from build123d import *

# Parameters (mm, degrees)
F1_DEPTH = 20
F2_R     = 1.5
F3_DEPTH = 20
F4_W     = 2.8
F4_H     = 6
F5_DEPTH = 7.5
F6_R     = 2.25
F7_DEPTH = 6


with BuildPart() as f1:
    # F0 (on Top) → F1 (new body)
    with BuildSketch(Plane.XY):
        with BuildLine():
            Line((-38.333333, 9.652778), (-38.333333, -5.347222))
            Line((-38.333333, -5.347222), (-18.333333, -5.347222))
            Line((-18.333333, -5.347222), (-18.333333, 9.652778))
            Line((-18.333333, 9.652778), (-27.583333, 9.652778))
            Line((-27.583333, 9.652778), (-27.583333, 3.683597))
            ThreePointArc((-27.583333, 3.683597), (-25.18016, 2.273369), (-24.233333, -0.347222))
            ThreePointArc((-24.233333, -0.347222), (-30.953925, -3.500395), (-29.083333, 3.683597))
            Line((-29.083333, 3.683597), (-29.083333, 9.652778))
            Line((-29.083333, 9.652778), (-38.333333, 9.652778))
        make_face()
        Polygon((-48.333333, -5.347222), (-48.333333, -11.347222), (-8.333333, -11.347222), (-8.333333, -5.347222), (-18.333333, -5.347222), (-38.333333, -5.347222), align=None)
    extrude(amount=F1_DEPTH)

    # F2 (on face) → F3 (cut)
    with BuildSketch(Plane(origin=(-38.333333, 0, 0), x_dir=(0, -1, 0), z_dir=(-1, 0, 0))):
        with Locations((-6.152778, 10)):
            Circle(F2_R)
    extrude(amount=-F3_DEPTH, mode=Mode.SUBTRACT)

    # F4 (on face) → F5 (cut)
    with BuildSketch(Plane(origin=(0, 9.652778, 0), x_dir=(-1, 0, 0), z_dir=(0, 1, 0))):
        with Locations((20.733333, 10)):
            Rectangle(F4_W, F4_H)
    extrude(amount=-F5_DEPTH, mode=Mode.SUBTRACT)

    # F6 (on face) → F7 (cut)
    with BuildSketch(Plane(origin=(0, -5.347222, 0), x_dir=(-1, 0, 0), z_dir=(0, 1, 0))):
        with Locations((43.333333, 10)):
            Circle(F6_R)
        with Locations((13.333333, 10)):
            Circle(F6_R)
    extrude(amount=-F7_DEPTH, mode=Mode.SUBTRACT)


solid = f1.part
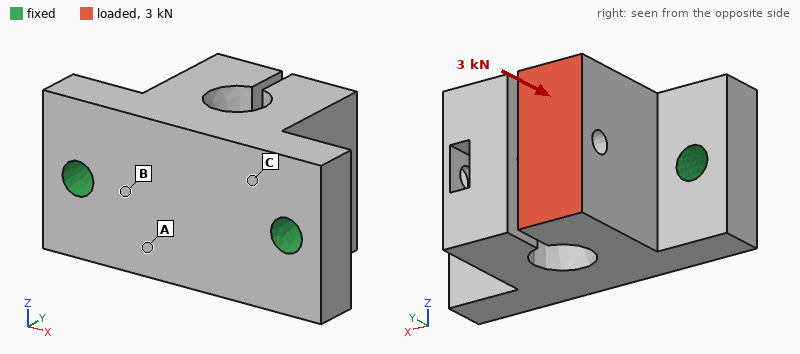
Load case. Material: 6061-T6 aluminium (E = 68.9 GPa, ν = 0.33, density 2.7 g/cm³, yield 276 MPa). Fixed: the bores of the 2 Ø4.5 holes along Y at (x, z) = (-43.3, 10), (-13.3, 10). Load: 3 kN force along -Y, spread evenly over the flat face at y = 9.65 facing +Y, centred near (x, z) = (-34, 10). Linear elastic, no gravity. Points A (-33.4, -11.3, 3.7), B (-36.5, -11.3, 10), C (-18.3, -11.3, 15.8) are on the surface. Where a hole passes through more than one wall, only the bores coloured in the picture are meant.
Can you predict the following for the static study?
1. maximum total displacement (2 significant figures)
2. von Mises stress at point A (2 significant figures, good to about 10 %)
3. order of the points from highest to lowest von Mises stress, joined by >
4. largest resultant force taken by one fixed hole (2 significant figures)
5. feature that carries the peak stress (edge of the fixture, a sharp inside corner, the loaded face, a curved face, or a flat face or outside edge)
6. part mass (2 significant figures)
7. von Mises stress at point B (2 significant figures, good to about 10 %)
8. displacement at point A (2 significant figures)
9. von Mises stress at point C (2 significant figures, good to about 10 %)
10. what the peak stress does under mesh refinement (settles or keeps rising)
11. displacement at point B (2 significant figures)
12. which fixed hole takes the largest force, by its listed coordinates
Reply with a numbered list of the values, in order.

1. 41 µm
2. 37 MPa
3. A > B > C
4. 2.2 kN
5. edge of the fixture
6. 25 g
7. 21 MPa
8. 13 µm
9. 11 MPa
10. keeps rising
11. 9.8 µm
12. (-43.3, 10)
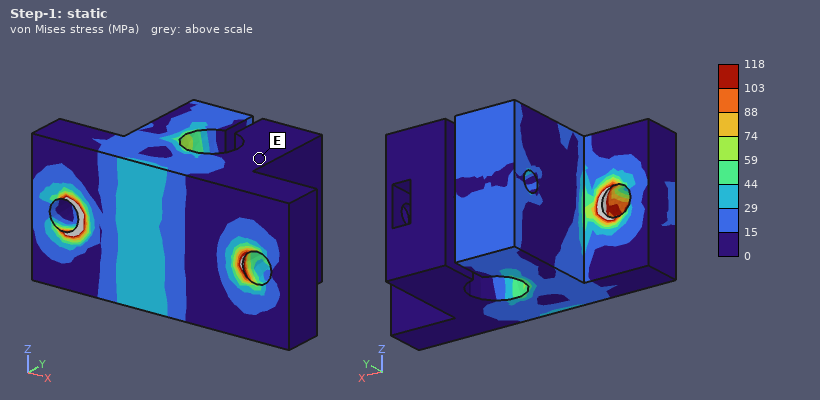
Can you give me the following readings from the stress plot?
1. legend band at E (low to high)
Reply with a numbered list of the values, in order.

1. 0 to 15 MPa
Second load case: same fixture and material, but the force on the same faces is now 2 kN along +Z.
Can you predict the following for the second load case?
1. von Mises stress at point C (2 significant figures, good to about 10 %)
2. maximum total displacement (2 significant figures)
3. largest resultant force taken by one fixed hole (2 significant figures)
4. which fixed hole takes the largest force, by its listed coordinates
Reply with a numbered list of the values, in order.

1. 42 MPa
2. 0.11 mm
3. 1.4 kN
4. (-43.3, 10)
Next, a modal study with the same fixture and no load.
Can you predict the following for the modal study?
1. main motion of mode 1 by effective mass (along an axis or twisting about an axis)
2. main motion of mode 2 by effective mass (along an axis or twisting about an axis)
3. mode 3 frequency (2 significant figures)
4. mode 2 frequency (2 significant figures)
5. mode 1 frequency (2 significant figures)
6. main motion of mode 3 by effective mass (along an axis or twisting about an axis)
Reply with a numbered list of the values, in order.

1. along Z
2. along Y
3. 15 kHz
4. 12 kHz
5. 9900 Hz
6. along X
